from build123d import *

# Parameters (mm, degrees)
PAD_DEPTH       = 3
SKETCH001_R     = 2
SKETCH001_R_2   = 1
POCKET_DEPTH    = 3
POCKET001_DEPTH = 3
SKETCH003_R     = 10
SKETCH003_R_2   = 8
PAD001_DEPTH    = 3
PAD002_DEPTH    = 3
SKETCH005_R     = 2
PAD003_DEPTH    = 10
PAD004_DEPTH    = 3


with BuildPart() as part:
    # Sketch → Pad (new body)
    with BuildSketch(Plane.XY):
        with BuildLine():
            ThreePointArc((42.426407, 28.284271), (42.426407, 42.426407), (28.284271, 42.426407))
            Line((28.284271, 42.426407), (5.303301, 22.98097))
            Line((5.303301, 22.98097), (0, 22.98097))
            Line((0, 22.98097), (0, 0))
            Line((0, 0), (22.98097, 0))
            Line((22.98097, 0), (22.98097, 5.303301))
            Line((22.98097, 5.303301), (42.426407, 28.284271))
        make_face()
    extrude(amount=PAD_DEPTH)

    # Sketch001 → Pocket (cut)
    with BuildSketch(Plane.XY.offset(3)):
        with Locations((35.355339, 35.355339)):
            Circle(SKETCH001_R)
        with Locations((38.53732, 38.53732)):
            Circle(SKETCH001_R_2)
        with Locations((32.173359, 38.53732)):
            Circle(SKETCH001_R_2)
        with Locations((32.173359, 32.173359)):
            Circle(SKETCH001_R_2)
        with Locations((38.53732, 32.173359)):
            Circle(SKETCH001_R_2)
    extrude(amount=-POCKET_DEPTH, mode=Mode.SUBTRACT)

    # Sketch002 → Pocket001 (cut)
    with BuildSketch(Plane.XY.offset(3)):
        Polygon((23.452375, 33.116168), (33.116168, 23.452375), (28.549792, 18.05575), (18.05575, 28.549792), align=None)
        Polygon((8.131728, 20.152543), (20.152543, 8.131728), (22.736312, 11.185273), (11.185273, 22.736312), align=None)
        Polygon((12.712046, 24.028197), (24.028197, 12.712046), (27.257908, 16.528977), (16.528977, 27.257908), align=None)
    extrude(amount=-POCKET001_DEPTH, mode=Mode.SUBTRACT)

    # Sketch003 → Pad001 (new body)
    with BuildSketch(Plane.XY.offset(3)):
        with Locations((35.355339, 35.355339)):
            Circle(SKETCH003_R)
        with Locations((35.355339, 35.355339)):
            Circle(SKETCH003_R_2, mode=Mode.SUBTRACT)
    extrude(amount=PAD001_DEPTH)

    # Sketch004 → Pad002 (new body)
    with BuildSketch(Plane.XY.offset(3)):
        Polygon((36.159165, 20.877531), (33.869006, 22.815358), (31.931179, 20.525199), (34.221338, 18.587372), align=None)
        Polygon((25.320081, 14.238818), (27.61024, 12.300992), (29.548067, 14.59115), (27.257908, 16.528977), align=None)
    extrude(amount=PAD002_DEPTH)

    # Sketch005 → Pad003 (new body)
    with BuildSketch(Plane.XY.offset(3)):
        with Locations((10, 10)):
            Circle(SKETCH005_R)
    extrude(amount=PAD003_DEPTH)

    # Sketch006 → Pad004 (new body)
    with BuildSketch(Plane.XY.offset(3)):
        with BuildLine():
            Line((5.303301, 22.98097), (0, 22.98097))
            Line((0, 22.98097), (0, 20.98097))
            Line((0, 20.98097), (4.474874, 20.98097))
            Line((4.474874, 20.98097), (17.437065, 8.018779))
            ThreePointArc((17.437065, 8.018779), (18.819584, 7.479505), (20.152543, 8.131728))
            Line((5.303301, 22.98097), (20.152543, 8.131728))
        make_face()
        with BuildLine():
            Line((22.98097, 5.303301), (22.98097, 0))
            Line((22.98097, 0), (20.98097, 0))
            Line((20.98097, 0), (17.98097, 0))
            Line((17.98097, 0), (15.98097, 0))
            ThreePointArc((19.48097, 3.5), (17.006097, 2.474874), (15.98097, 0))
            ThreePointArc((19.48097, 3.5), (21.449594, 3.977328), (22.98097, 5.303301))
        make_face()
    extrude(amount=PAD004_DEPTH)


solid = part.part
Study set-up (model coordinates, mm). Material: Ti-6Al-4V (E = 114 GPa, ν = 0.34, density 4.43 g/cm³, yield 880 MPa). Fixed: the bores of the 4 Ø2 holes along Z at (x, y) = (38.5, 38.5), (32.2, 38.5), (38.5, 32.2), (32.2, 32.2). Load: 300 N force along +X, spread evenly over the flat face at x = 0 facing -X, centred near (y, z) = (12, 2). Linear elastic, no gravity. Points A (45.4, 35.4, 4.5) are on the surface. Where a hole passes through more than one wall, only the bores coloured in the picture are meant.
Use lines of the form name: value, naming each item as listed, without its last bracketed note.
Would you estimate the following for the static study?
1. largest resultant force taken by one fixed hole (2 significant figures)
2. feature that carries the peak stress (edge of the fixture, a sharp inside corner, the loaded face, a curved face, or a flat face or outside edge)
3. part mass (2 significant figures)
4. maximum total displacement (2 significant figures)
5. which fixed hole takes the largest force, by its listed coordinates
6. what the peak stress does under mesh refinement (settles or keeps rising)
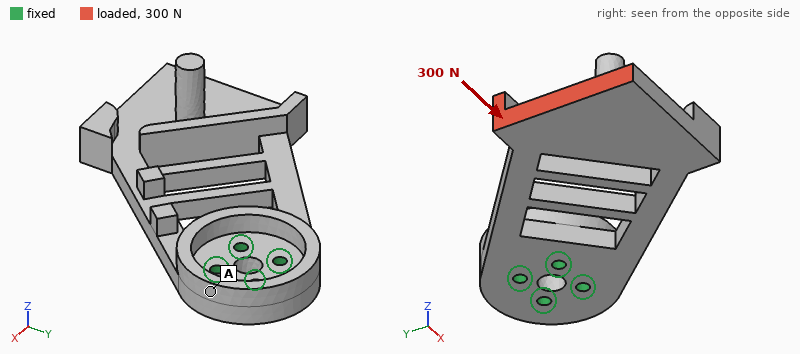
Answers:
largest resultant force taken by one fixed hole: 500 N
feature that carries the peak stress: a sharp inside corner
part mass: 16 g
maximum total displacement: 93 µm
which fixed hole takes the largest force, by its listed coordinates: (32.2, 32.2)
what the peak stress does under mesh refinement: keeps rising
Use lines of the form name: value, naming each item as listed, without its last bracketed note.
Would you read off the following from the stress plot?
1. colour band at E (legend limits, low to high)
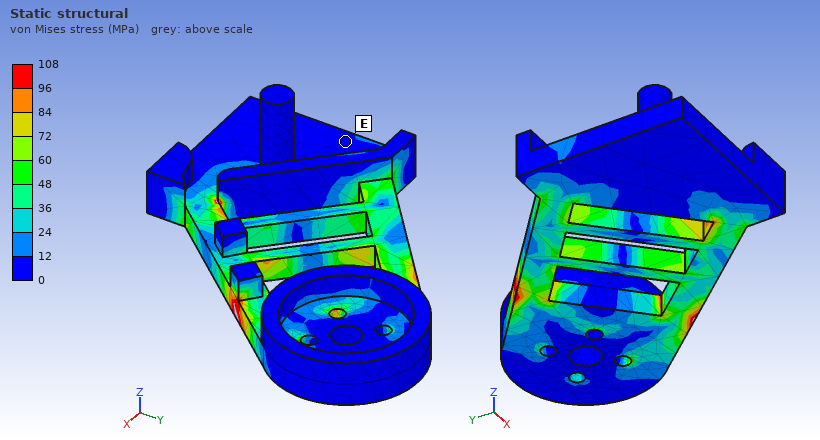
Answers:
colour band at E: 0 to 12 MPa
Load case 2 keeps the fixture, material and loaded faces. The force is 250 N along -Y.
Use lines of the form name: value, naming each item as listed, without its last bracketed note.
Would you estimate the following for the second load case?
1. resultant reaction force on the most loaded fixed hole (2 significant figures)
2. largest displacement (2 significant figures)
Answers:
resultant reaction force on the most loaded fixed hole: 560 N
largest displacement: 0.10 mm
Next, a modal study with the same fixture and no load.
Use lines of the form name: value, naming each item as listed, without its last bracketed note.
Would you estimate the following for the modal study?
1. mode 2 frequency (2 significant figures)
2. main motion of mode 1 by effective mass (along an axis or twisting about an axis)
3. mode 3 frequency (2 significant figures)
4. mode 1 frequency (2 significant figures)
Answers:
mode 2 frequency: 2800 Hz
main motion of mode 1 by effective mass: along Z
mode 3 frequency: 3100 Hz
mode 1 frequency: 890 Hz
